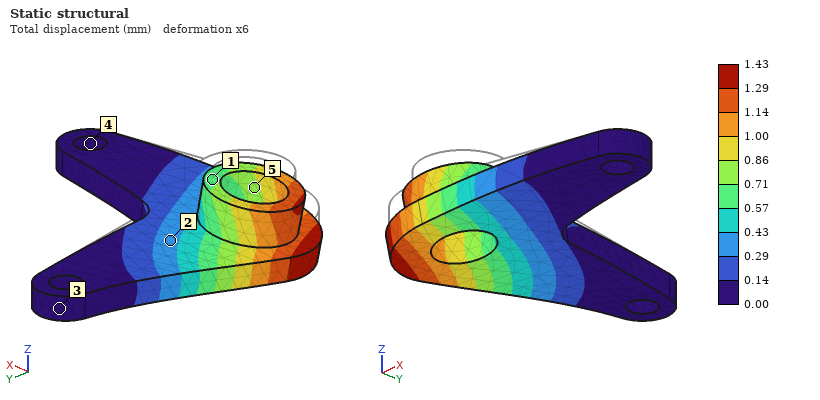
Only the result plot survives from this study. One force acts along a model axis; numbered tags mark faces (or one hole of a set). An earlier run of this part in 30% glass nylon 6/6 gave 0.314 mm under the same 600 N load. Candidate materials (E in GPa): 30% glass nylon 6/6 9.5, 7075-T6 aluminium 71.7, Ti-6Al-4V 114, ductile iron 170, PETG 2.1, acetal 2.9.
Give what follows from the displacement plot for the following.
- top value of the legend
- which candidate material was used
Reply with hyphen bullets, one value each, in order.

- 1.43 mm
- PETG
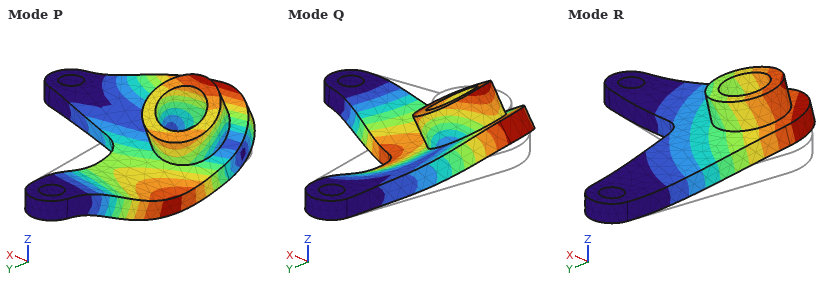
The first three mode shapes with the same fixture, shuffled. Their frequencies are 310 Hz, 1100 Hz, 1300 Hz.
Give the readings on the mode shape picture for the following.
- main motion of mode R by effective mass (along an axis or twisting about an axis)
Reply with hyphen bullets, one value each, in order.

- along Z
